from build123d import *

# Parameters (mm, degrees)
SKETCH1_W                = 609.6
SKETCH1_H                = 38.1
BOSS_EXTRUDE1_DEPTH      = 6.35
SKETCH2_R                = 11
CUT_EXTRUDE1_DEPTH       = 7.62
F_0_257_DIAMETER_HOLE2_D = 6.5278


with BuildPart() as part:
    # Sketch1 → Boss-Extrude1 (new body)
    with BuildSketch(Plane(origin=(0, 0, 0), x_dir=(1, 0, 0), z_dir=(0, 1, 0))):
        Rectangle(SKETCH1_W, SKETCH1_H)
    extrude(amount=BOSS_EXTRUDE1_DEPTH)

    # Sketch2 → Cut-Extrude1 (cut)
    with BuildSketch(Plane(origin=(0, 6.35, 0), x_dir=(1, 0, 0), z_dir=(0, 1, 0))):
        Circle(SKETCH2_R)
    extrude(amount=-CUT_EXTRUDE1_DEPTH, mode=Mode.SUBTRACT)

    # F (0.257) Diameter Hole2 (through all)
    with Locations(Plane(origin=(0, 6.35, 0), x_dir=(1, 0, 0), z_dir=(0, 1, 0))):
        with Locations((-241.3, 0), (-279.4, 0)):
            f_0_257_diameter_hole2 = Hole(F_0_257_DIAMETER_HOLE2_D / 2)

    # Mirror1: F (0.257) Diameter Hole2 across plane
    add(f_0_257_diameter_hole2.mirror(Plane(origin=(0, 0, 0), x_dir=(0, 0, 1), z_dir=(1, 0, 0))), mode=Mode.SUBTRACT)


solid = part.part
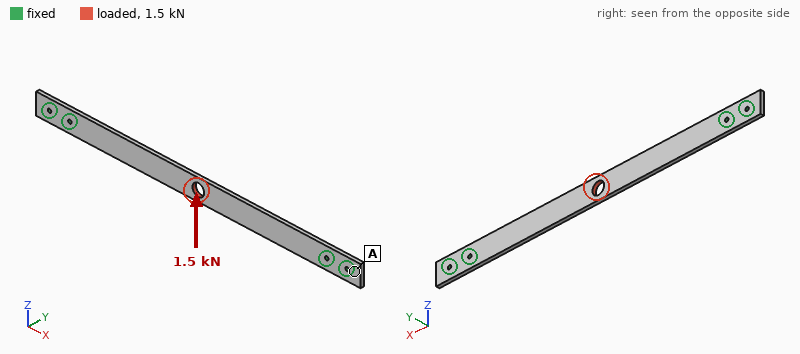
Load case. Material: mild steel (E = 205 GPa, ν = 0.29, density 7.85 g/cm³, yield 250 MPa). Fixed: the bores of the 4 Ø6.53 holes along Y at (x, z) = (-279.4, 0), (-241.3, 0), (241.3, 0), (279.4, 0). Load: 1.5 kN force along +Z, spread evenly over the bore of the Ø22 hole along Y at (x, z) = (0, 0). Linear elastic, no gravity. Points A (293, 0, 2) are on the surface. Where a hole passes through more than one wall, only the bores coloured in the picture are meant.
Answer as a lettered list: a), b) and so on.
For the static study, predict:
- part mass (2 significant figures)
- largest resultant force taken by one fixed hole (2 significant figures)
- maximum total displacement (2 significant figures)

a) 1.1 kg
b) 2.5 kN
c) 0.19 mm
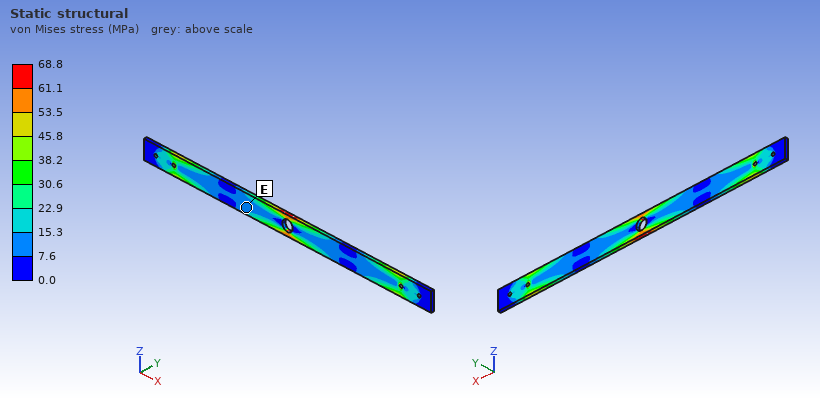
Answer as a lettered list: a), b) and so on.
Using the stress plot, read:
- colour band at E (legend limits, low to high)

a) 7.6 to 15.3 MPa
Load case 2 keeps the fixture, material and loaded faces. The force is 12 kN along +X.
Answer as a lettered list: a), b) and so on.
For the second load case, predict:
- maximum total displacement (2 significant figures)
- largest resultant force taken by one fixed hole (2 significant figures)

a) 30 µm
b) 4.9 kN
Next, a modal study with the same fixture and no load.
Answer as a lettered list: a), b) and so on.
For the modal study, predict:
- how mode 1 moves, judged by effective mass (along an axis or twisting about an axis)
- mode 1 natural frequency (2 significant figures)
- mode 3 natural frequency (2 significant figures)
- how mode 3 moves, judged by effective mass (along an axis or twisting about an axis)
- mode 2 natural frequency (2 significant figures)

a) along Y
b) 140 Hz
c) 750 Hz
d) along Z
e) 390 Hz
